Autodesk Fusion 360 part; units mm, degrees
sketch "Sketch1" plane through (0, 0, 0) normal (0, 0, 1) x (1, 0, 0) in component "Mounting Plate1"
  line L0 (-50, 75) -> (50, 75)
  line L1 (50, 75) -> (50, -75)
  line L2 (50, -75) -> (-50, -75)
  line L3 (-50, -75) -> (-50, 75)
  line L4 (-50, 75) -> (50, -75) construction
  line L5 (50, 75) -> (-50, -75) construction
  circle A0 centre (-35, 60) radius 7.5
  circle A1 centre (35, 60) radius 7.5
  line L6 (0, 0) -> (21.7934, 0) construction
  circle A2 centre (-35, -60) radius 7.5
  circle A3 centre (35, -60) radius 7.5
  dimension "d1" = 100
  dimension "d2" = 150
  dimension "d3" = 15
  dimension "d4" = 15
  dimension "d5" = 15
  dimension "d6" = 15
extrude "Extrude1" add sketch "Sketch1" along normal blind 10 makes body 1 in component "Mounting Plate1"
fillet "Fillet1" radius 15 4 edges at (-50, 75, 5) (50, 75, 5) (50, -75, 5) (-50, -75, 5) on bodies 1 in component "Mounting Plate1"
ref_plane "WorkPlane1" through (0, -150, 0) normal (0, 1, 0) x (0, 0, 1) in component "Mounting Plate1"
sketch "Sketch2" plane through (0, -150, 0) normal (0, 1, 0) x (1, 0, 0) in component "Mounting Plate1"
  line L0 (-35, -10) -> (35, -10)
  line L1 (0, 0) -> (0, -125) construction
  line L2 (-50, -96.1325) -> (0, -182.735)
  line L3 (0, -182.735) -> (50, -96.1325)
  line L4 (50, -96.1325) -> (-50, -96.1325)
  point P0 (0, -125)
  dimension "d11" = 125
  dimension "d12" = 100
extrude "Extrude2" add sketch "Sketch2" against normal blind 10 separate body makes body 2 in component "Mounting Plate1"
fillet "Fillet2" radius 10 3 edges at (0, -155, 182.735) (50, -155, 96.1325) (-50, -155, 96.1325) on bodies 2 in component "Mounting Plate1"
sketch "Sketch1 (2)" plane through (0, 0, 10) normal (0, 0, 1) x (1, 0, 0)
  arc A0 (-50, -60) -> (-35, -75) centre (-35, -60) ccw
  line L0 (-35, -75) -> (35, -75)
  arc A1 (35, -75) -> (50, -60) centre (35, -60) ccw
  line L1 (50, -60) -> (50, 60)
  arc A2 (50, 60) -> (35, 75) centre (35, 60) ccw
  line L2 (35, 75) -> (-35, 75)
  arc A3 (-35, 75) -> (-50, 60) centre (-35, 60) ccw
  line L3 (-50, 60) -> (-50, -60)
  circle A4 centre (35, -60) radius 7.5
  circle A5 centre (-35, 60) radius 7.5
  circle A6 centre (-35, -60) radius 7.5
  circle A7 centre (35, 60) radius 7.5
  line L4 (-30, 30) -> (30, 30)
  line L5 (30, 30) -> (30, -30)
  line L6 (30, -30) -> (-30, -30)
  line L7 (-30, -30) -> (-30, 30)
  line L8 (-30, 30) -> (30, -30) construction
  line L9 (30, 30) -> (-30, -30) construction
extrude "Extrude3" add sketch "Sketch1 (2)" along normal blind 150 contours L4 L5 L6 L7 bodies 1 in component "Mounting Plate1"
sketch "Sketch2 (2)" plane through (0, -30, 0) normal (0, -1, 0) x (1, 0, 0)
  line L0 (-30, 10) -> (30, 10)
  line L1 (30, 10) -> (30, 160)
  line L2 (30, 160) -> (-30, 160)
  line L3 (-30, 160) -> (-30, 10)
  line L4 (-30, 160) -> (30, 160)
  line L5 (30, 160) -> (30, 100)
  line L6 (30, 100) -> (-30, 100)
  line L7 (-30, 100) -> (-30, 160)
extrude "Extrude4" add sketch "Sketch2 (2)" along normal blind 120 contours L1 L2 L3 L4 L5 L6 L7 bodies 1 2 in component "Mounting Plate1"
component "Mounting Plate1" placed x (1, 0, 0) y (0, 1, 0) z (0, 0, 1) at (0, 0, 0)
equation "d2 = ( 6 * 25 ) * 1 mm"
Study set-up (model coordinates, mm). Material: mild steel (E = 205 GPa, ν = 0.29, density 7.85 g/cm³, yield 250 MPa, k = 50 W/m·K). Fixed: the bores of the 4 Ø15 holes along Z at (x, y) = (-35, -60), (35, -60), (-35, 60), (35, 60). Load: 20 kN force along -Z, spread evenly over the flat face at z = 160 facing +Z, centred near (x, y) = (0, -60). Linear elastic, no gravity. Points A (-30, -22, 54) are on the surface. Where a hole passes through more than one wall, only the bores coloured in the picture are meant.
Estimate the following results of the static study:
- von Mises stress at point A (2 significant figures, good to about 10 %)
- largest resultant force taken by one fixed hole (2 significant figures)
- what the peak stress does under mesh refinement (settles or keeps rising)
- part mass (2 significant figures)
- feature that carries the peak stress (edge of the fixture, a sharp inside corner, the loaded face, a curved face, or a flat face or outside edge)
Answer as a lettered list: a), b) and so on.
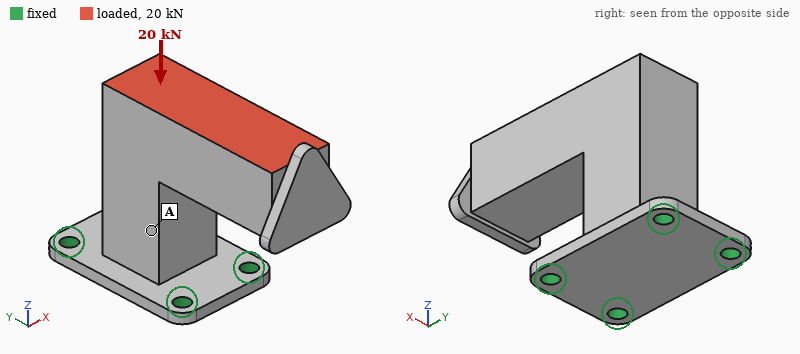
a) 30 MPa
b) 12 kN
c) keeps rising
d) 9.1 kg
e) edge of the fixture
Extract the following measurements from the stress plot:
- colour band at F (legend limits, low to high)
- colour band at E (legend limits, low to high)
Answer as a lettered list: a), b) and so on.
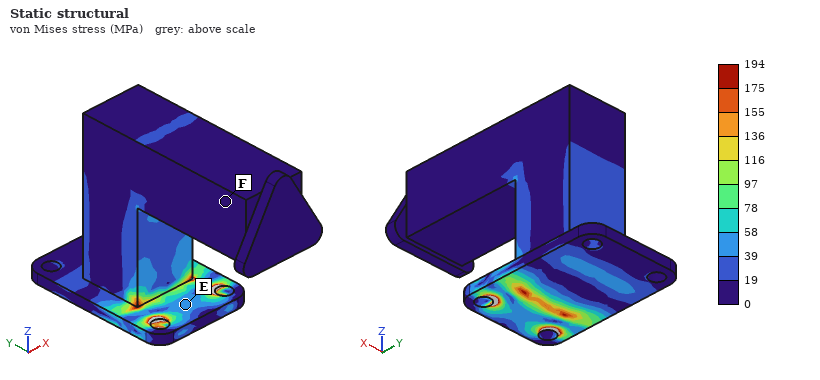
a) 0 to 19 MPa
b) 39 to 58 MPa
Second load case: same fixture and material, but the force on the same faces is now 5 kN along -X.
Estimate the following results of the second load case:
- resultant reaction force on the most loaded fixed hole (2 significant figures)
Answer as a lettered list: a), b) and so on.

a) 6.4 kN
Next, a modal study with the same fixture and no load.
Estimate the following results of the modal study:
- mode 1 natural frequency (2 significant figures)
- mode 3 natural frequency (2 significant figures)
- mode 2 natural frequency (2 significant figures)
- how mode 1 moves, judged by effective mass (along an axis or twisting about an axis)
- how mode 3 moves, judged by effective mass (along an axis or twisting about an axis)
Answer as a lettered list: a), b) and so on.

a) 370 Hz
b) 1200 Hz
c) 420 Hz
d) along X
e) twisting about Z
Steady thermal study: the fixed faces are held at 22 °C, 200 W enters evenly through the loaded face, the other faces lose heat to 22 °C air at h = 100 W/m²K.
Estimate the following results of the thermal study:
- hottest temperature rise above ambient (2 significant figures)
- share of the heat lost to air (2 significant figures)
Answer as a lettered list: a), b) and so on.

a) 49 K
b) 93 %
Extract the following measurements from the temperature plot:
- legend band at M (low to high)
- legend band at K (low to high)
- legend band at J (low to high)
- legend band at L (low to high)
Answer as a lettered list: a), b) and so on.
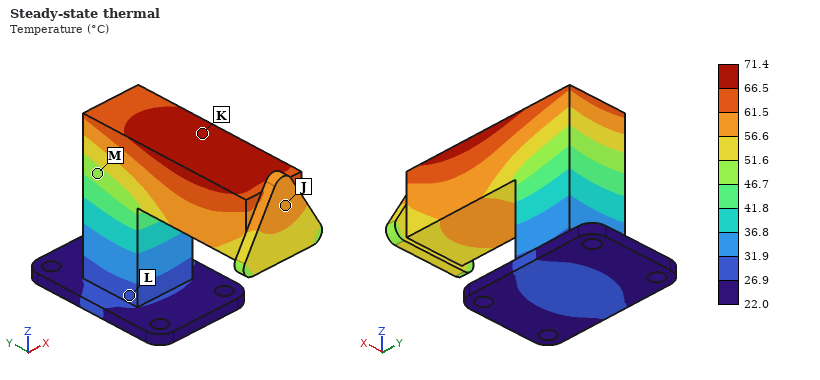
a) 46.7 to 51.6 °C
b) 66.5 to 71.4 °C
c) 56.6 to 61.5 °C
d) 26.9 to 31.9 °C
